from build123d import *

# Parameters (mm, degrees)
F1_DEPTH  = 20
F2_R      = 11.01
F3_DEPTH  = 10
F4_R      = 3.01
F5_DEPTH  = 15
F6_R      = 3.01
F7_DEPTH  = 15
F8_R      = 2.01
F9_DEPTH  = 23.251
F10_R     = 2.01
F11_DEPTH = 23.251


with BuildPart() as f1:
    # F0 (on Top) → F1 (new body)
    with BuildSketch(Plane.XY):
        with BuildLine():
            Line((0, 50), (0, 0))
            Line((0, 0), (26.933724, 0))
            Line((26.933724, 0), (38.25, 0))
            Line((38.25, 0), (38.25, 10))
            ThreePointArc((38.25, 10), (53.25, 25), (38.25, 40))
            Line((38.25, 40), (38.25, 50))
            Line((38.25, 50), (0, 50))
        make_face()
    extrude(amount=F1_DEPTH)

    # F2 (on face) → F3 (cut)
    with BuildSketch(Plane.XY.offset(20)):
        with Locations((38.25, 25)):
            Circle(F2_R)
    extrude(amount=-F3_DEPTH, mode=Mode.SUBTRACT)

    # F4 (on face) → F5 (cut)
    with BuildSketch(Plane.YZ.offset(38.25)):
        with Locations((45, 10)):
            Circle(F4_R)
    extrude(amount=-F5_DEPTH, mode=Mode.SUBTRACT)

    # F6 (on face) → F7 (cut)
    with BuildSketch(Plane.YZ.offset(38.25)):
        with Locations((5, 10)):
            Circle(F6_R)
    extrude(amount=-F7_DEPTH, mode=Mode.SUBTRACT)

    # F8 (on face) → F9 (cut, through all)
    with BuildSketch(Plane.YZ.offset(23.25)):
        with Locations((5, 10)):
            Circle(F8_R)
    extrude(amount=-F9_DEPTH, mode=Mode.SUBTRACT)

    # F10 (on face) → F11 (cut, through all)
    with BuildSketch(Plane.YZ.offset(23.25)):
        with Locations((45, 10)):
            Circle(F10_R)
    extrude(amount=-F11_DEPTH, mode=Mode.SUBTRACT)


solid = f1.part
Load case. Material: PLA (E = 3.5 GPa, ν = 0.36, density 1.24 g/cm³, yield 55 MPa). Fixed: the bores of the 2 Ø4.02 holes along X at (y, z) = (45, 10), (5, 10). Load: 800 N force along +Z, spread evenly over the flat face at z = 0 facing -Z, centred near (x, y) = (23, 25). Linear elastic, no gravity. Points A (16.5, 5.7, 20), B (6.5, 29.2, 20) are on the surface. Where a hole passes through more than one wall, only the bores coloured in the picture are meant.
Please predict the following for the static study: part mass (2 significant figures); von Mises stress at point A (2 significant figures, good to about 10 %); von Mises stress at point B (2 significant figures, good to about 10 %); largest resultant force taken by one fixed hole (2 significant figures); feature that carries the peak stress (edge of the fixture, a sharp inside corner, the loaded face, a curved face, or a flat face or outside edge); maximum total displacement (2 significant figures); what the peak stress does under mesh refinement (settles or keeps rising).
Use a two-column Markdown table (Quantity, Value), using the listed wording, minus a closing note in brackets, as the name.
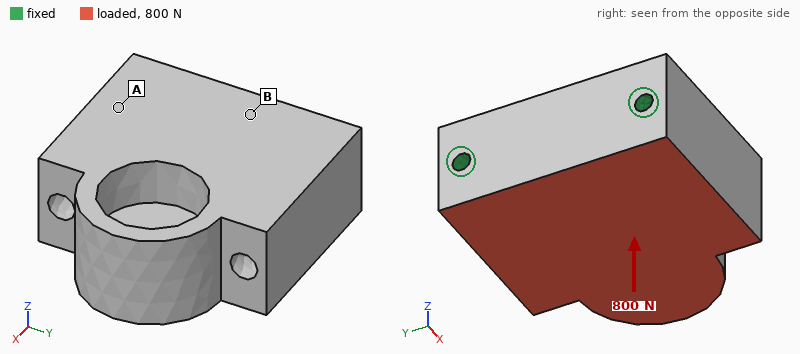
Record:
| Quantity | Value |
|---|---|
| part mass | 50 g |
| von Mises stress at point A | 2.1 MPa |
| von Mises stress at point B | 0.92 MPa |
| largest resultant force taken by one fixed hole | 400 N |
| feature that carries the peak stress | edge of the fixture |
| maximum total displacement | 84 µm |
| what the peak stress does under mesh refinement | keeps rising |
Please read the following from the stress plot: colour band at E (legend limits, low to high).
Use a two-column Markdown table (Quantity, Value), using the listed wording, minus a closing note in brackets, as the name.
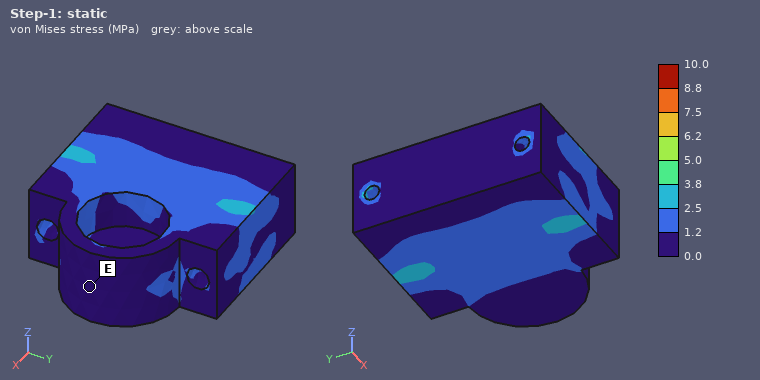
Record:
| Quantity | Value |
|---|---|
| colour band at E | 0.0 to 1.2 MPa |
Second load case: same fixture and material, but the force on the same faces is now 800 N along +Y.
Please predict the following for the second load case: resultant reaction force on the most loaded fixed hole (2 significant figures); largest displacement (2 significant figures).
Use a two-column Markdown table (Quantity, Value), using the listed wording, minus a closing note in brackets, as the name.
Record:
| Quantity | Value |
|---|---|
| resultant reaction force on the most loaded fixed hole | 470 N |
| largest displacement | 21 µm |
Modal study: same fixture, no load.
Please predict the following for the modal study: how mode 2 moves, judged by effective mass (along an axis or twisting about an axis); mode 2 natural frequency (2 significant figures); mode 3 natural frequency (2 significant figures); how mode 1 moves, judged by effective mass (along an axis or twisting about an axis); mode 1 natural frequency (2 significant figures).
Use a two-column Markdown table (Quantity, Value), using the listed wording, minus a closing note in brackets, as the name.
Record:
| Quantity | Value |
|---|---|
| how mode 2 moves, judged by effective mass | along Y |
| mode 2 natural frequency | 6000 Hz |
| mode 3 natural frequency | 7300 Hz |
| how mode 1 moves, judged by effective mass | along Z |
| mode 1 natural frequency | 3200 Hz |
